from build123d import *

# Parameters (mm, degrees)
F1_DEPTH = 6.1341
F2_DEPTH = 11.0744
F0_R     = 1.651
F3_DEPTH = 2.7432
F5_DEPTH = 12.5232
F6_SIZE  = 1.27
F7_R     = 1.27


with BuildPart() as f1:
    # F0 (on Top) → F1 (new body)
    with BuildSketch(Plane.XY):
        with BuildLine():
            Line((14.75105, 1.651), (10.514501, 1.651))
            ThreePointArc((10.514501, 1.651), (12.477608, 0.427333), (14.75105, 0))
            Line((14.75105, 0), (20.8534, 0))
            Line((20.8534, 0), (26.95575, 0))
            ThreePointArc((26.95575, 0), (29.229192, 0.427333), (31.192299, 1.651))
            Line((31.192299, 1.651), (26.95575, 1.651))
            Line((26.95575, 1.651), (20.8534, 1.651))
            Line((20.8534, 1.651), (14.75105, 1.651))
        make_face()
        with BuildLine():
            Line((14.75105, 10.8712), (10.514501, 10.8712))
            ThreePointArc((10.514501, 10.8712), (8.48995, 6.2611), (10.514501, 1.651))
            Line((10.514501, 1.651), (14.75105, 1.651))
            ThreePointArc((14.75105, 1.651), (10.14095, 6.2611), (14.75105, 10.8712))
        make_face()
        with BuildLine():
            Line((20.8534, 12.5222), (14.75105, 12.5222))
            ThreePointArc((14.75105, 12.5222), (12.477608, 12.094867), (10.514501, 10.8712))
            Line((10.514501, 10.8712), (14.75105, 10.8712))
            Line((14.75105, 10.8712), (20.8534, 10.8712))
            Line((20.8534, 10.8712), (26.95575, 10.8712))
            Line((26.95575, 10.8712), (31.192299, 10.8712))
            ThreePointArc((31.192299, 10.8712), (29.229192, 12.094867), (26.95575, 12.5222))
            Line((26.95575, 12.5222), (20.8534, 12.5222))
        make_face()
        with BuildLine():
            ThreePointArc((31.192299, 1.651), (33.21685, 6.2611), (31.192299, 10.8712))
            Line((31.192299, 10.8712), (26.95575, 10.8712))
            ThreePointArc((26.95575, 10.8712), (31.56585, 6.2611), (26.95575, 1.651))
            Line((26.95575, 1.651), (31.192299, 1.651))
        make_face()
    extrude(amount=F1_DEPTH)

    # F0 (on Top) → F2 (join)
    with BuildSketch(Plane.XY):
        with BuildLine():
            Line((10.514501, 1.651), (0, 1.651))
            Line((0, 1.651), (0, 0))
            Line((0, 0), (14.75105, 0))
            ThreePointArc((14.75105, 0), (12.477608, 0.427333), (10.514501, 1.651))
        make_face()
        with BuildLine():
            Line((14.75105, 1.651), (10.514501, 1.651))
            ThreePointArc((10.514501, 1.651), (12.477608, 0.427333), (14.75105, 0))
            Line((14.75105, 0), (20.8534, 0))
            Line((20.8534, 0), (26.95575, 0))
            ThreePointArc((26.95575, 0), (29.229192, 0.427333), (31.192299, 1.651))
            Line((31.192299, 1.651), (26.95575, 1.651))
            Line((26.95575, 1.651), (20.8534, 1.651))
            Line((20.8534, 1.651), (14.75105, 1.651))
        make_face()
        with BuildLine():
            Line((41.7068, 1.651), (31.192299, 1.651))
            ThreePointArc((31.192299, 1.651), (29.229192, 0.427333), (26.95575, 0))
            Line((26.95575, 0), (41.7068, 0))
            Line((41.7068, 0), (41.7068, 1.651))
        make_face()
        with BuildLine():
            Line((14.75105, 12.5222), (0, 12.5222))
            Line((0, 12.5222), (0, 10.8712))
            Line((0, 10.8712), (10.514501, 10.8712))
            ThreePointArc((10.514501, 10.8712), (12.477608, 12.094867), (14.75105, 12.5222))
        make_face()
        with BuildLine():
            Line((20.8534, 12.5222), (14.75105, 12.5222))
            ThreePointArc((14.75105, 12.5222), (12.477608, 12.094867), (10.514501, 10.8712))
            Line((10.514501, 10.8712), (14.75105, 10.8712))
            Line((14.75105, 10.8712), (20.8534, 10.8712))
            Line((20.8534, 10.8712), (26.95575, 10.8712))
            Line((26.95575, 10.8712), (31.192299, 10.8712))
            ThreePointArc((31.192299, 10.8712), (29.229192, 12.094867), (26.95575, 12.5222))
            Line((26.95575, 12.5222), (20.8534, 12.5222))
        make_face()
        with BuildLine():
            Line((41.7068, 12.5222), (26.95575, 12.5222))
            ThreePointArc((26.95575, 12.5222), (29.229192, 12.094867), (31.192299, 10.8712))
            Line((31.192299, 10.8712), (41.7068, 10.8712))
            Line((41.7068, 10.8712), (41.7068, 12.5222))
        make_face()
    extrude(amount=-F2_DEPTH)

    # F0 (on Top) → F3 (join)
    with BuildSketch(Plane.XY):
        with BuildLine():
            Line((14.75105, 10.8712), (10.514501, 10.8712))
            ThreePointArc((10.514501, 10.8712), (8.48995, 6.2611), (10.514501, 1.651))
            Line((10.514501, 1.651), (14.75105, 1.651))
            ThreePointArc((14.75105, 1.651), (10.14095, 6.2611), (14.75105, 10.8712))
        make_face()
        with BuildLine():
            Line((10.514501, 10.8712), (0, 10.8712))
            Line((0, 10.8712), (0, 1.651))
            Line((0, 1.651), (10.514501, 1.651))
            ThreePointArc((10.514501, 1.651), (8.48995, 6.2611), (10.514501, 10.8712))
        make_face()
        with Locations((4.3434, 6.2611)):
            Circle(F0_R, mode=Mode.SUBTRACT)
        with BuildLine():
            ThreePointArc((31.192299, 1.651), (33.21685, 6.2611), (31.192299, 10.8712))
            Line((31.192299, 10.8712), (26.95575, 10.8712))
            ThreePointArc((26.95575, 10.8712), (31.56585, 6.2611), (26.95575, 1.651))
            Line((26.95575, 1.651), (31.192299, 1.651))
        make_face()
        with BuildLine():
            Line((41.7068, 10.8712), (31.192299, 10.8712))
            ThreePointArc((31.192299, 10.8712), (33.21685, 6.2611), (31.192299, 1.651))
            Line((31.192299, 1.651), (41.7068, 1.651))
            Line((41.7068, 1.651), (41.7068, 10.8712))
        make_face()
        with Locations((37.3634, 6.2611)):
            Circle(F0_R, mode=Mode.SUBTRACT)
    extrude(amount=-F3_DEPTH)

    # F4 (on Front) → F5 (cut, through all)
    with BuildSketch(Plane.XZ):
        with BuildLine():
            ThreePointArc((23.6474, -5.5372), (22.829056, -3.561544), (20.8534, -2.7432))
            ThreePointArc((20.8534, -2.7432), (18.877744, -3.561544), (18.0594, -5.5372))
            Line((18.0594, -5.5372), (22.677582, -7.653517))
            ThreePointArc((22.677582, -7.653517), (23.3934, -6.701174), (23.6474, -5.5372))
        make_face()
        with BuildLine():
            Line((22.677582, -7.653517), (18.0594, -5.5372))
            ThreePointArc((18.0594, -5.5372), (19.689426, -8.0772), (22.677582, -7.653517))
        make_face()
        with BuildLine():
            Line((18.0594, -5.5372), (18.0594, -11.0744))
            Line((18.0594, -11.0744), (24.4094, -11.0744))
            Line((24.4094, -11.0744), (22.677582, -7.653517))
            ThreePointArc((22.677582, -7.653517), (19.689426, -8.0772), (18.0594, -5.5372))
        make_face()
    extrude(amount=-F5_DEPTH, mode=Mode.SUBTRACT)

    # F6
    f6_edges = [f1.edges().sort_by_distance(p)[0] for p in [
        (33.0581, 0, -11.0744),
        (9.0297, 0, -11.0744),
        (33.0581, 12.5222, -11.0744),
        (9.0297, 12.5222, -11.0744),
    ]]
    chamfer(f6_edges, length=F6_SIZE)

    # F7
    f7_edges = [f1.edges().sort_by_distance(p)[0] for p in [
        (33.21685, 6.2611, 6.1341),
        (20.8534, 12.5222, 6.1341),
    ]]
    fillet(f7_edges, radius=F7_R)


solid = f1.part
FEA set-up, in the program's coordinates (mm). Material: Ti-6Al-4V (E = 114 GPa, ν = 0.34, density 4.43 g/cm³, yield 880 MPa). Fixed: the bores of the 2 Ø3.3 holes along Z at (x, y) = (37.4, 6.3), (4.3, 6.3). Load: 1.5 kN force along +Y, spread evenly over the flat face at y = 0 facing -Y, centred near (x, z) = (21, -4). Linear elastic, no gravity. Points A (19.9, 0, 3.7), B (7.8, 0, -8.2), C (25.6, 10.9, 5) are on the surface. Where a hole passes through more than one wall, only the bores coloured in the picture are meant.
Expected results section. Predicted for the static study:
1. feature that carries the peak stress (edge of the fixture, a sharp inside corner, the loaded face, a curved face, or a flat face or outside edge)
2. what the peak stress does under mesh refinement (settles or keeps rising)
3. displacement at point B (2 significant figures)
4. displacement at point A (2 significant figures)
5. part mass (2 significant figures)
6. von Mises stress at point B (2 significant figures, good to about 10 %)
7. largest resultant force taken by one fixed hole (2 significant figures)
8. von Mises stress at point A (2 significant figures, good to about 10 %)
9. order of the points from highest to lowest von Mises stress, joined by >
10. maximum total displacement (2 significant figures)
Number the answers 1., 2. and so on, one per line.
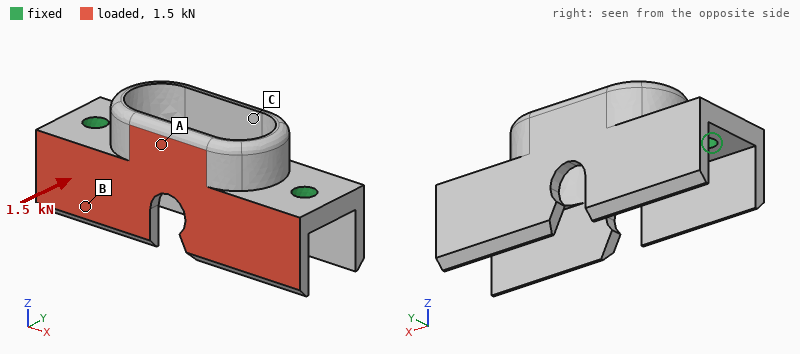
1. a sharp inside corner
2. keeps rising
3. 0.052 mm
4. 0.020 mm
5. 11 g
6. 48 MPa
7. 810 N
8. 96 MPa
9. A > B > C
10. 0.12 mm
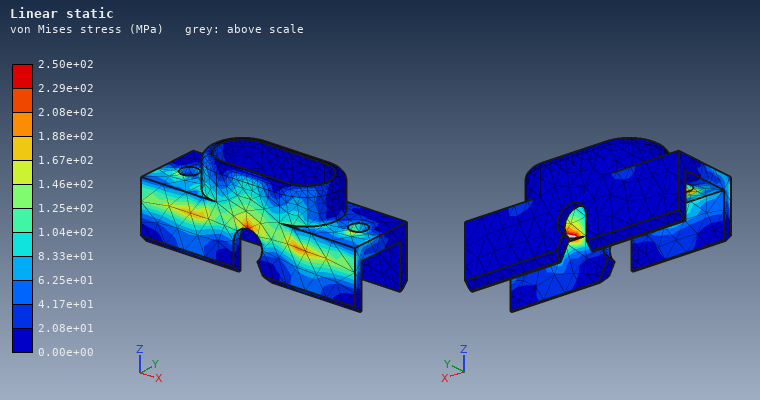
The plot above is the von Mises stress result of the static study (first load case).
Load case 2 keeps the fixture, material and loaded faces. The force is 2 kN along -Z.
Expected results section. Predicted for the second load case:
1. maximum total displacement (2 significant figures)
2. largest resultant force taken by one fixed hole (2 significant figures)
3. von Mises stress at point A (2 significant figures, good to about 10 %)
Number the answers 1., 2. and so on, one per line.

1. 0.11 mm
2. 1.0 kN
3. 53 MPa
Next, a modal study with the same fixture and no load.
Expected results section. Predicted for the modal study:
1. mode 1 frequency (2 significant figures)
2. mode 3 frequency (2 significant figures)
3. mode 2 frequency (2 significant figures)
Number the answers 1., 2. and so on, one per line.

1. 11 kHz
2. 13 kHz
3. 13 kHz
